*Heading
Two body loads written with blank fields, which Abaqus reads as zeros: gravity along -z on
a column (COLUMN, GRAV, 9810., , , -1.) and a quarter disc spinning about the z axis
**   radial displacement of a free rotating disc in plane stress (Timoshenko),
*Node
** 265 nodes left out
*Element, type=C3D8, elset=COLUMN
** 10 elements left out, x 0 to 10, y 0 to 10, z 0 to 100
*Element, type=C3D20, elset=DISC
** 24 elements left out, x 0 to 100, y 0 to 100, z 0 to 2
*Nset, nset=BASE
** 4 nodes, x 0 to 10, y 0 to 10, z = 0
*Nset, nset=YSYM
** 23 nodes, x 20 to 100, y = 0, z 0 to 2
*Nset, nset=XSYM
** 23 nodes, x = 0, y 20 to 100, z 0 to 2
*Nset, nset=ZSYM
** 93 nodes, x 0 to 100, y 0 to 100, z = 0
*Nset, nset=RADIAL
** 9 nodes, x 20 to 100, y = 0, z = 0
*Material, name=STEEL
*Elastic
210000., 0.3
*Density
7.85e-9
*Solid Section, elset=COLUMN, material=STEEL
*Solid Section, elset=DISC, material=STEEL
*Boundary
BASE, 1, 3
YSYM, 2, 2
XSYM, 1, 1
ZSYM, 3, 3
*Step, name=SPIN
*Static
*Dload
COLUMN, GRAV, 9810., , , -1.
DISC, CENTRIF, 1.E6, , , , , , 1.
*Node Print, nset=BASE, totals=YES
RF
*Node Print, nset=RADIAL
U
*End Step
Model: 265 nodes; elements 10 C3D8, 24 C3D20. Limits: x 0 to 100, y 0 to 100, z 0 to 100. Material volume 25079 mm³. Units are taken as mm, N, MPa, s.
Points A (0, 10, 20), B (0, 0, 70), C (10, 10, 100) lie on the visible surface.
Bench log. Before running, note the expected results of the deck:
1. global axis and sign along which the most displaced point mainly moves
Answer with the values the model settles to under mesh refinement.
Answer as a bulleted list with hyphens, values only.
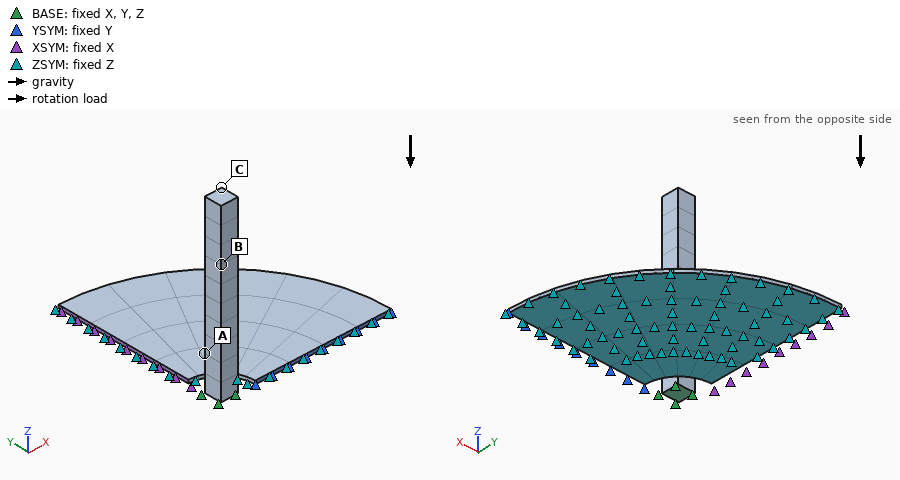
- +X
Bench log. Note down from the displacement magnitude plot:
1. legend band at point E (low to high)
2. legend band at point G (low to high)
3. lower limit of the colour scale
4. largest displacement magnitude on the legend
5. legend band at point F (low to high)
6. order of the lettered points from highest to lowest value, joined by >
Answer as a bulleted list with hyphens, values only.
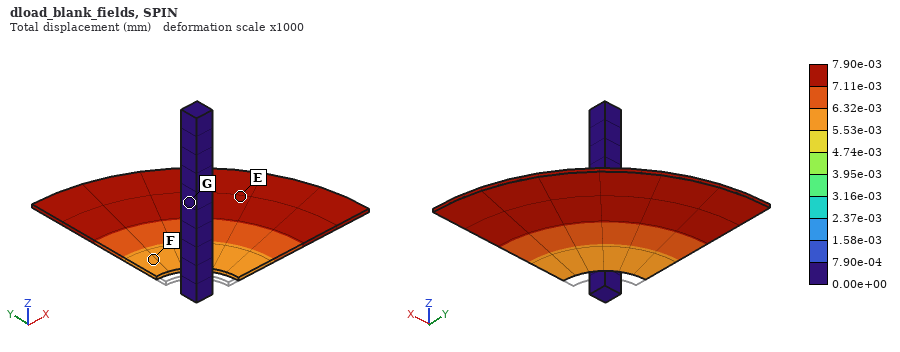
- 7.11e-03 to 7.90e-03 mm
- 0.00e+00 to 7.90e-04 mm
- 0.00e+00 mm
- 7.90e-03 mm
- 5.53e-03 to 6.32e-03 mm
- E > F > G
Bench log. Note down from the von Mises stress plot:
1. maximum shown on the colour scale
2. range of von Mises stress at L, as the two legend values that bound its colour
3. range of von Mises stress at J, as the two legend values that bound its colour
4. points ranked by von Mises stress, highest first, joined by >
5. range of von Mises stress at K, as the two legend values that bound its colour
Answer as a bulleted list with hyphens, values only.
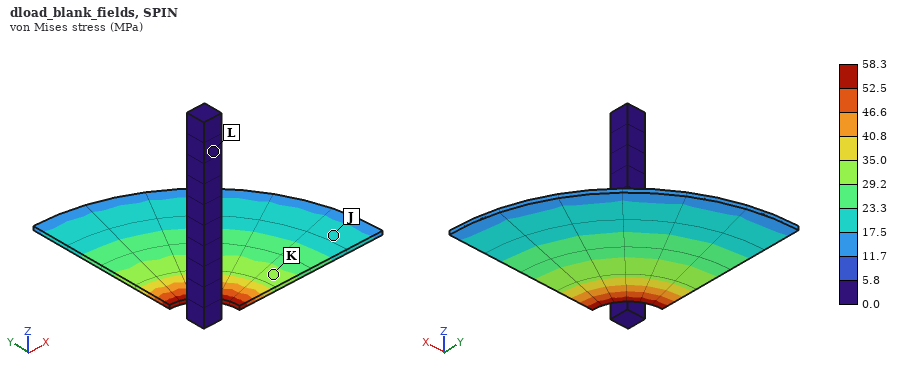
- 58.3 MPa
- 0.0 to 5.8 MPa
- 17.5 to 23.3 MPa
- K > J > L
- 29.2 to 35.0 MPa
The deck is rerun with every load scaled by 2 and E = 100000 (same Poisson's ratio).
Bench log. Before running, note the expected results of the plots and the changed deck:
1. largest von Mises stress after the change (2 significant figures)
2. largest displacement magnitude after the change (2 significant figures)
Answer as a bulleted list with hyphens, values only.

- 120 MPa
- 0.033 mm
